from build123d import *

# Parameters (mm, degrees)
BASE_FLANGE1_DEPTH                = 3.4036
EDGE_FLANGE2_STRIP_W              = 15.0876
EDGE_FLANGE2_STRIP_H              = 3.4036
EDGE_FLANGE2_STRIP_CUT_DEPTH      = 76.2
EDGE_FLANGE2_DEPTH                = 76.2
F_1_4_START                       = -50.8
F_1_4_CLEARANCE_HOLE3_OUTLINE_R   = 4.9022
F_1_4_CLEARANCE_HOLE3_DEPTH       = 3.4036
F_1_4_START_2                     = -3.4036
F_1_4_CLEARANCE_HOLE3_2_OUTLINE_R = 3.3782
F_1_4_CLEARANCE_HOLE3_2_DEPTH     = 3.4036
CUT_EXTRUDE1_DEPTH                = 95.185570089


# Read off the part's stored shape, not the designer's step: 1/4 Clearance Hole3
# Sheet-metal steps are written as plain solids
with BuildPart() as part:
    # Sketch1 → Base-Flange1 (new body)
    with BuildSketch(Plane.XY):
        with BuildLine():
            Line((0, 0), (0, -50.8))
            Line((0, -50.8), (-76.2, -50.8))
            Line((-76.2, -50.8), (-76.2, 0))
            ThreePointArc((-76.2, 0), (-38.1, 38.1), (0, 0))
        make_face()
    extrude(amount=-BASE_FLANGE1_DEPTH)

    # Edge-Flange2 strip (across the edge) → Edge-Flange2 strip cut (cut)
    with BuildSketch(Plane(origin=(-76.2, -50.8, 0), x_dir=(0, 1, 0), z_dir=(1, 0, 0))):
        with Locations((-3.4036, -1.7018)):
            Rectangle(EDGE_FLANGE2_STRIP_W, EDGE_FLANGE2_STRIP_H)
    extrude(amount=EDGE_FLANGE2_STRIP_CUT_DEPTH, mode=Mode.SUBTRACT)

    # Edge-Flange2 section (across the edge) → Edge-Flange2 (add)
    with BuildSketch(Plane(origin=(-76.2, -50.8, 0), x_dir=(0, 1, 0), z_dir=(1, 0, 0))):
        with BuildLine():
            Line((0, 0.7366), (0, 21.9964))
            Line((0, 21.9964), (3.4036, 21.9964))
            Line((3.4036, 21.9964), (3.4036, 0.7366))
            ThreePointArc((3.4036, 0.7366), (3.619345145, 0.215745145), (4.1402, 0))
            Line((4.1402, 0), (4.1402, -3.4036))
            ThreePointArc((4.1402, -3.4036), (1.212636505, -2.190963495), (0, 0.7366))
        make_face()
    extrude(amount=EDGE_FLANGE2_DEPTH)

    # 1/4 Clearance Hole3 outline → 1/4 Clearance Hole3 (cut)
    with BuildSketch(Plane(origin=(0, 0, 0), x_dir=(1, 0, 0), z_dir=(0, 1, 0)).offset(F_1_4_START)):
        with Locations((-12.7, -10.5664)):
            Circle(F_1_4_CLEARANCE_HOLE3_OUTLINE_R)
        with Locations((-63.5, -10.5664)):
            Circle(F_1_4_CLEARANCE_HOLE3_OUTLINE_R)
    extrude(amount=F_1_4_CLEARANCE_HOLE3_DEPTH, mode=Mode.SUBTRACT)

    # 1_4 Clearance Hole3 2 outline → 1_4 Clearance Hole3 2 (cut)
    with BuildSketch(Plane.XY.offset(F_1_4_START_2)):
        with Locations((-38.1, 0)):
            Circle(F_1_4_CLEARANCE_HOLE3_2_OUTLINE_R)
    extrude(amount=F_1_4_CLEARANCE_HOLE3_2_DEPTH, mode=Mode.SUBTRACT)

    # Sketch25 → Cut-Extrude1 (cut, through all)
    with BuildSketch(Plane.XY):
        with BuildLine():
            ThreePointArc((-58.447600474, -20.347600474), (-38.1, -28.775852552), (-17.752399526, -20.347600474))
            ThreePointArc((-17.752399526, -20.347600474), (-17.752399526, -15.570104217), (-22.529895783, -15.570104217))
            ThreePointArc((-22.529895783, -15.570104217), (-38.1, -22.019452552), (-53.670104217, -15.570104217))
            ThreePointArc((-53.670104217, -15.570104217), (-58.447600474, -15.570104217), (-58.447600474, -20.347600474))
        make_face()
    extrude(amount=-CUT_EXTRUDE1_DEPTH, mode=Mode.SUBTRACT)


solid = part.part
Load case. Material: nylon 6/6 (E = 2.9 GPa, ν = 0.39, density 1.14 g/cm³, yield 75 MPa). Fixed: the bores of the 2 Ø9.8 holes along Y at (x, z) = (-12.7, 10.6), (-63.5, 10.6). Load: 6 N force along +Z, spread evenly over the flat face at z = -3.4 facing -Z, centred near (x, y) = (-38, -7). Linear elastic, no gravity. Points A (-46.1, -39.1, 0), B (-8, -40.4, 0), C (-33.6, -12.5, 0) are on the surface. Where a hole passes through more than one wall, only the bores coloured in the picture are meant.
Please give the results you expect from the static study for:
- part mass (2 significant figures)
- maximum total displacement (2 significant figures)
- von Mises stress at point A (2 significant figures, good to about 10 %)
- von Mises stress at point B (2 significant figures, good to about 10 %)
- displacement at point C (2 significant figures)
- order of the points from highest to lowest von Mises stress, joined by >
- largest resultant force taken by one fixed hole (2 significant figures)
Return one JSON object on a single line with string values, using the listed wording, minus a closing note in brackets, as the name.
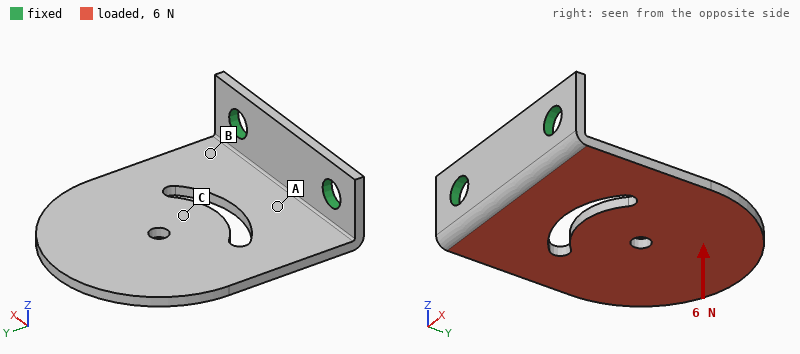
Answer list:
{"part mass": "28 g", "maximum total displacement": "1.1 mm", "von Mises stress at point A": "1.0 MPa", "von Mises stress at point B": "1.4 MPa", "displacement at point C": "0.31 mm", "order of the points from highest to lowest von Mises stress, joined by >": "B > A > C", "largest resultant force taken by one fixed hole": "3.0 N"}
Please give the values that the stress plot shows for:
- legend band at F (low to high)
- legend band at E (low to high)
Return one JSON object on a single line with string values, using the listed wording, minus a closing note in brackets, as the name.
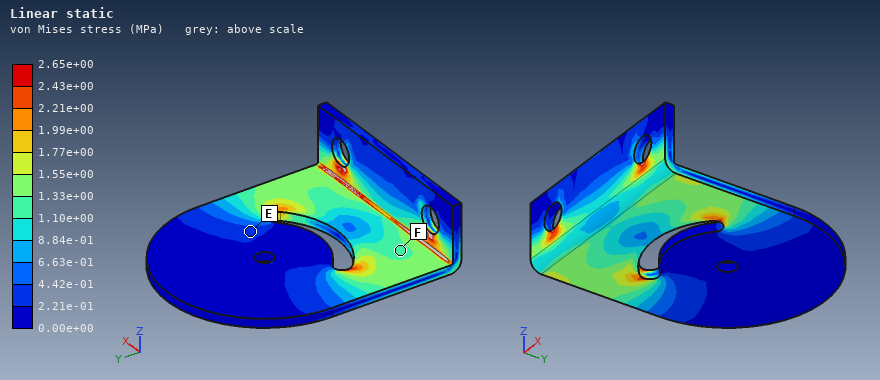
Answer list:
{"legend band at F": "1.10e+00 to 1.33e+00 MPa", "legend band at E": "2.21e-01 to 4.42e-01 MPa"}
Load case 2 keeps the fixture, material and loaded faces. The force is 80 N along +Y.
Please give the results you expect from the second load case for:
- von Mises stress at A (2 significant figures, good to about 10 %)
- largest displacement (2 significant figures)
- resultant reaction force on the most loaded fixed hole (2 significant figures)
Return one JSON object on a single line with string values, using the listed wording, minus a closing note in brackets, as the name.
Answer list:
{"von Mises stress at A": "0.82 MPa", "largest displacement": "1.2 mm", "resultant reaction force on the most loaded fixed hole": "40 N"}
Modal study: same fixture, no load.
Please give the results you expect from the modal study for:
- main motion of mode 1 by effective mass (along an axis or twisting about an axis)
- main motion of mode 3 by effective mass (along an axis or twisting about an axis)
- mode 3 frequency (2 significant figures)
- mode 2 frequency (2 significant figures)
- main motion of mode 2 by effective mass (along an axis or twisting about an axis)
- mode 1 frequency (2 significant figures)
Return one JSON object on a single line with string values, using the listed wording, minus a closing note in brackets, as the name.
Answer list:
{"main motion of mode 1 by effective mass": "along Z", "main motion of mode 3 by effective mass": "along Z", "mode 3 frequency": "600 Hz", "mode 2 frequency": "340 Hz", "main motion of mode 2 by effective mass": "twisting about Y", "mode 1 frequency": "100 Hz"}
